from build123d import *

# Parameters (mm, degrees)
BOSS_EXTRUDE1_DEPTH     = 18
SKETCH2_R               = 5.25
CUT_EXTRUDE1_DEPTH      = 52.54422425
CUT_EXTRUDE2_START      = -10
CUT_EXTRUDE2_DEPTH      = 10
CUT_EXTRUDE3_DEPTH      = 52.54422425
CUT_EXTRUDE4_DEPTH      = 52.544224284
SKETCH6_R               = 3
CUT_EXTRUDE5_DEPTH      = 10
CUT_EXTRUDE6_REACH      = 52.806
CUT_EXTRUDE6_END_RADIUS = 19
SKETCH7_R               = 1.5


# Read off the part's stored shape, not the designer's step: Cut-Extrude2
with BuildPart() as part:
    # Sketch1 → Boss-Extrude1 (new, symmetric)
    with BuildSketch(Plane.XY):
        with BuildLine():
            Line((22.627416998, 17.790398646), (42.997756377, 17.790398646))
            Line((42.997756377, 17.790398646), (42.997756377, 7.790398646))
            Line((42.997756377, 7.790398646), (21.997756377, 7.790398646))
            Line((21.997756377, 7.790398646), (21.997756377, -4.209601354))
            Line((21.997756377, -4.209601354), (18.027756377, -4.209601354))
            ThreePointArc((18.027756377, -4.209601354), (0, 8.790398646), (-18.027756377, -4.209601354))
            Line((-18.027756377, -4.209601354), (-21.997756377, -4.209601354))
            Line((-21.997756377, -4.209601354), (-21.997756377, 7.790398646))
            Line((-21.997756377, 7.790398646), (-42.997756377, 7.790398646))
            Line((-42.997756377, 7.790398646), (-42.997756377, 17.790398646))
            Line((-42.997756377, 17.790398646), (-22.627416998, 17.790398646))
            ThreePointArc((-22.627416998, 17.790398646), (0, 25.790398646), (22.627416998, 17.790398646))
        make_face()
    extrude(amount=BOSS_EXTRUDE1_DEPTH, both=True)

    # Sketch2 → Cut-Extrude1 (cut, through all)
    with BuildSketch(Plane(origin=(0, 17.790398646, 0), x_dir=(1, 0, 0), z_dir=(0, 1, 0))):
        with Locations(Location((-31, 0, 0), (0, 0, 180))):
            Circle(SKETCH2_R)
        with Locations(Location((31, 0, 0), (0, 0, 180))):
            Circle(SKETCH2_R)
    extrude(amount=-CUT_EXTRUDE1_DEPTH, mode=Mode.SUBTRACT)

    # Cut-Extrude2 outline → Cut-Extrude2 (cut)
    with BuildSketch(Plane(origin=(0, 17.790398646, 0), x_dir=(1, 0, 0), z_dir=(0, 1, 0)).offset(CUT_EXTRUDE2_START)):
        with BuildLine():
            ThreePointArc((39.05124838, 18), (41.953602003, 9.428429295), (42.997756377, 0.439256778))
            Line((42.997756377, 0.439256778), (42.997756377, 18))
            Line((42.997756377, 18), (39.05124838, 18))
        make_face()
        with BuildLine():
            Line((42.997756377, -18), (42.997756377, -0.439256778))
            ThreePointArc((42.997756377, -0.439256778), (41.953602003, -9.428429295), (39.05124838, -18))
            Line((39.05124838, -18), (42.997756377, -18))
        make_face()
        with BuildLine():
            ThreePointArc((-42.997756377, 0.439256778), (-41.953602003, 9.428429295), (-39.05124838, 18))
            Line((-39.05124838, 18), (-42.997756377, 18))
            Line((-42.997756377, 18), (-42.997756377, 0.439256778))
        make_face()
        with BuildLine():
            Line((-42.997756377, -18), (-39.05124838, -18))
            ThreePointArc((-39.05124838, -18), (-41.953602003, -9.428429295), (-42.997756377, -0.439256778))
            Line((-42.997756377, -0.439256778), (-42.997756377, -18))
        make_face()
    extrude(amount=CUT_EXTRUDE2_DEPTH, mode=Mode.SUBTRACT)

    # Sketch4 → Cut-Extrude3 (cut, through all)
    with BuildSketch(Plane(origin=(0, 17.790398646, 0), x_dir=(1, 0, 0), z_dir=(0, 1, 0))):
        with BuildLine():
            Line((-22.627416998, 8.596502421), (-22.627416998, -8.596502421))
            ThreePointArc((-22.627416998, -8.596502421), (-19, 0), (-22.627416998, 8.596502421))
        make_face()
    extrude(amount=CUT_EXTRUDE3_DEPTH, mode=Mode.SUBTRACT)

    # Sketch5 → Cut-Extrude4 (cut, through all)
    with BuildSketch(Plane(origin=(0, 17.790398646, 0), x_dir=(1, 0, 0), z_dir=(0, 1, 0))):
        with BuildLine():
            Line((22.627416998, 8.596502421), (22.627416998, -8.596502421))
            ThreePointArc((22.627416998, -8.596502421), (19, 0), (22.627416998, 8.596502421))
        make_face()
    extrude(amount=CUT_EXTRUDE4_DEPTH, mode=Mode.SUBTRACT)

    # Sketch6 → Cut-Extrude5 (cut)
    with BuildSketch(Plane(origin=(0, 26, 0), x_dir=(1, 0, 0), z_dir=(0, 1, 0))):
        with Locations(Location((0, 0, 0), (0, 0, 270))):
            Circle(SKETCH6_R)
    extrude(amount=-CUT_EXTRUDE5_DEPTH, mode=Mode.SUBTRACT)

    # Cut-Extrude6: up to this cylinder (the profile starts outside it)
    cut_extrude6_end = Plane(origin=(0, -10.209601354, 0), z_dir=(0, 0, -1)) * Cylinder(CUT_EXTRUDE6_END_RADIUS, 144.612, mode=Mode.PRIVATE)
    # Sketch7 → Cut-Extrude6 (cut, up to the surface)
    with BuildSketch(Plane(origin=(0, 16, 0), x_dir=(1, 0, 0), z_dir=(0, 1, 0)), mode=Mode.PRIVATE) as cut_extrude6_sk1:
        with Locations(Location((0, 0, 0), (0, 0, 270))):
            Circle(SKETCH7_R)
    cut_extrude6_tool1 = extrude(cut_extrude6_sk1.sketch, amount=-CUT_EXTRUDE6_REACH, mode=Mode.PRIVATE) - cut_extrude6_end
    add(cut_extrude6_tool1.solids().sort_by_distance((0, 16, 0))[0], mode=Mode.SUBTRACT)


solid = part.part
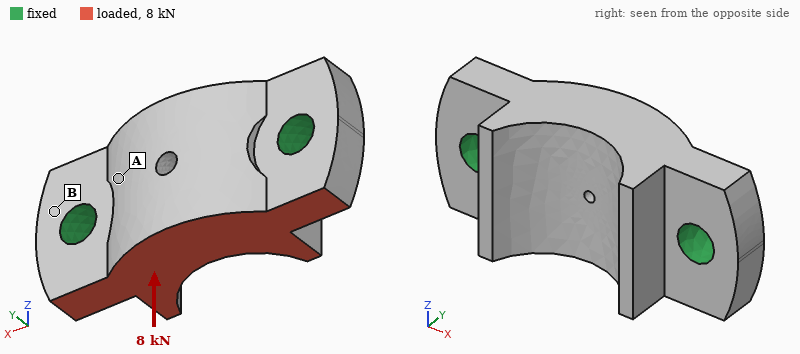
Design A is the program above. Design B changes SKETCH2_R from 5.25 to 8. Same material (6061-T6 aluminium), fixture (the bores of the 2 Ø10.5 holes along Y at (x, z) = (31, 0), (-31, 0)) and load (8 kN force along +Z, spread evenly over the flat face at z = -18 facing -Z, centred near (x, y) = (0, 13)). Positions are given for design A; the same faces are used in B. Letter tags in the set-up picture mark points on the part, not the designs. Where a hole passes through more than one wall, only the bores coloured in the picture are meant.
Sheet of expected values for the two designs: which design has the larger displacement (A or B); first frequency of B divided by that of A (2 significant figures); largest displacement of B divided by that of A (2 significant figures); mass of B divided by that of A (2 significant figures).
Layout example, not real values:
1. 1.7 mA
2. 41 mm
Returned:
1. A
2. 1.3
3. 0.75
4. 0.95
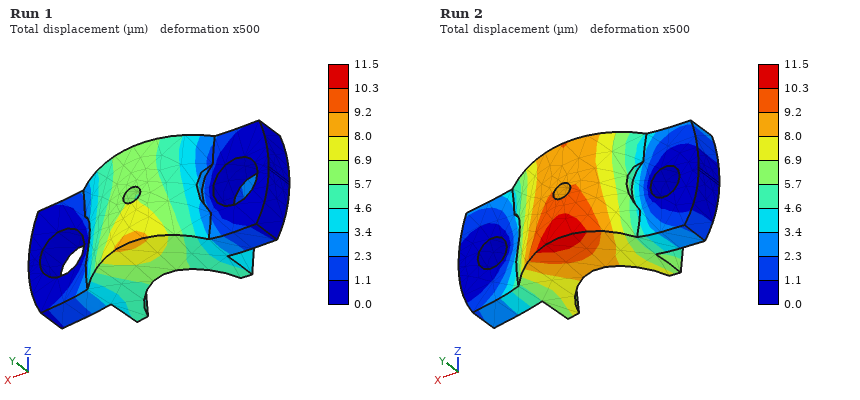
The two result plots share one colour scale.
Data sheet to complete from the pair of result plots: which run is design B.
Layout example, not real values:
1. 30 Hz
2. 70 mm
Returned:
1. Run 1
